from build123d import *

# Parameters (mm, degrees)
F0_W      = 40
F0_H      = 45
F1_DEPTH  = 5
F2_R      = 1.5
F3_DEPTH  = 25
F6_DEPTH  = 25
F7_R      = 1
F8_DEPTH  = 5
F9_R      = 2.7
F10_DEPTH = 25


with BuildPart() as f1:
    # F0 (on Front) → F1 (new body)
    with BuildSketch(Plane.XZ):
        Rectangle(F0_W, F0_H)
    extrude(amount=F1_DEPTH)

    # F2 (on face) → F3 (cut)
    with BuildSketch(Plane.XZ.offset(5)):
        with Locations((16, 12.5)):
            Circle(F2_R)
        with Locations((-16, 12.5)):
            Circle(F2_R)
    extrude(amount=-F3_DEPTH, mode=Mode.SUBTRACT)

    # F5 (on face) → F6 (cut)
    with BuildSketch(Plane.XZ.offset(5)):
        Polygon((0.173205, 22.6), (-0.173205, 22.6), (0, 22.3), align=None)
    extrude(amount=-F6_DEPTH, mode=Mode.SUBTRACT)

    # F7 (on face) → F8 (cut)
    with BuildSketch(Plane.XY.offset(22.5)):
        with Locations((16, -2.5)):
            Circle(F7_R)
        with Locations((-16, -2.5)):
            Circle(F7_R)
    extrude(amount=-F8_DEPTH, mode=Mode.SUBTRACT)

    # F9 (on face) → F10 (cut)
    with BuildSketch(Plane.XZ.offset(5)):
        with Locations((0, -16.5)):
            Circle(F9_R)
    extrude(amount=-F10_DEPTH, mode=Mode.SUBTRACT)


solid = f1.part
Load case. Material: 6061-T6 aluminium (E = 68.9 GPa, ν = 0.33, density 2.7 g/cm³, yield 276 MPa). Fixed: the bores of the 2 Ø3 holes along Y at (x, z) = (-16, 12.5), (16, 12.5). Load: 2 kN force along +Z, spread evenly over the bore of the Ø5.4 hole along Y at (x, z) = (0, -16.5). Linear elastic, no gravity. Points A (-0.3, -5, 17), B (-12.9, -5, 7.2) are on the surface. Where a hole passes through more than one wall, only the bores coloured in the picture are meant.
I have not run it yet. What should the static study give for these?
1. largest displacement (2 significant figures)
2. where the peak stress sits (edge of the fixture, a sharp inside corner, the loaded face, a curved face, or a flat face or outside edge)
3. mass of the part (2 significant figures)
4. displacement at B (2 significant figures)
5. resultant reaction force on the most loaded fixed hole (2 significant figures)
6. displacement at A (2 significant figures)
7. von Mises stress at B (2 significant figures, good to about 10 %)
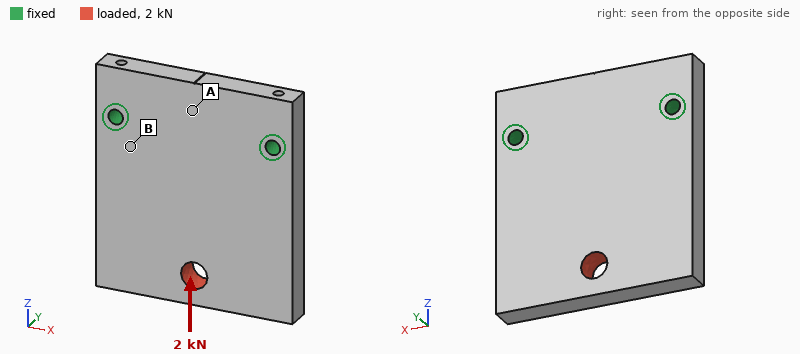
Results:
12 µm
the loaded face
24 g
1.8 µm
1.0 kN
3.1 µm
18 MPa
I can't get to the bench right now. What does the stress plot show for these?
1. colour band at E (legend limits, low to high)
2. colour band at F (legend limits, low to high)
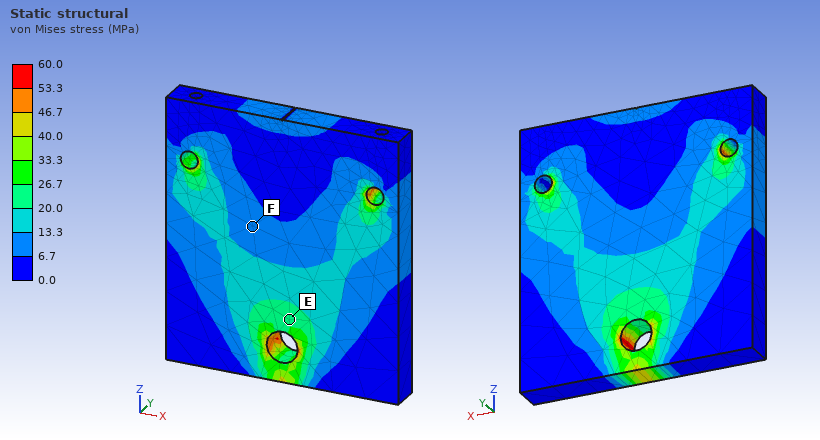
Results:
20.0 to 26.7 MPa
6.7 to 13.3 MPa
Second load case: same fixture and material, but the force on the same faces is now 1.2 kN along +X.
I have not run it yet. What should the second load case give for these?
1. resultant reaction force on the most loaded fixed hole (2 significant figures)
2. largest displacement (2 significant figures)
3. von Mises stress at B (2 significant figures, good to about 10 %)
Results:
1.2 kN
17 µm
21 MPa
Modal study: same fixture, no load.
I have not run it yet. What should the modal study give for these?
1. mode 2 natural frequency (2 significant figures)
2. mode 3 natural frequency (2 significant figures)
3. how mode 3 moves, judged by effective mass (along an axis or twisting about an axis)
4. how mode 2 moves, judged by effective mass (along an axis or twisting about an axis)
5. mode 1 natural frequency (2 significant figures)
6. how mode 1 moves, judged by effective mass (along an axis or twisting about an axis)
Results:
6900 Hz
15 kHz
along X
twisting about Z
2900 Hz
along Y
